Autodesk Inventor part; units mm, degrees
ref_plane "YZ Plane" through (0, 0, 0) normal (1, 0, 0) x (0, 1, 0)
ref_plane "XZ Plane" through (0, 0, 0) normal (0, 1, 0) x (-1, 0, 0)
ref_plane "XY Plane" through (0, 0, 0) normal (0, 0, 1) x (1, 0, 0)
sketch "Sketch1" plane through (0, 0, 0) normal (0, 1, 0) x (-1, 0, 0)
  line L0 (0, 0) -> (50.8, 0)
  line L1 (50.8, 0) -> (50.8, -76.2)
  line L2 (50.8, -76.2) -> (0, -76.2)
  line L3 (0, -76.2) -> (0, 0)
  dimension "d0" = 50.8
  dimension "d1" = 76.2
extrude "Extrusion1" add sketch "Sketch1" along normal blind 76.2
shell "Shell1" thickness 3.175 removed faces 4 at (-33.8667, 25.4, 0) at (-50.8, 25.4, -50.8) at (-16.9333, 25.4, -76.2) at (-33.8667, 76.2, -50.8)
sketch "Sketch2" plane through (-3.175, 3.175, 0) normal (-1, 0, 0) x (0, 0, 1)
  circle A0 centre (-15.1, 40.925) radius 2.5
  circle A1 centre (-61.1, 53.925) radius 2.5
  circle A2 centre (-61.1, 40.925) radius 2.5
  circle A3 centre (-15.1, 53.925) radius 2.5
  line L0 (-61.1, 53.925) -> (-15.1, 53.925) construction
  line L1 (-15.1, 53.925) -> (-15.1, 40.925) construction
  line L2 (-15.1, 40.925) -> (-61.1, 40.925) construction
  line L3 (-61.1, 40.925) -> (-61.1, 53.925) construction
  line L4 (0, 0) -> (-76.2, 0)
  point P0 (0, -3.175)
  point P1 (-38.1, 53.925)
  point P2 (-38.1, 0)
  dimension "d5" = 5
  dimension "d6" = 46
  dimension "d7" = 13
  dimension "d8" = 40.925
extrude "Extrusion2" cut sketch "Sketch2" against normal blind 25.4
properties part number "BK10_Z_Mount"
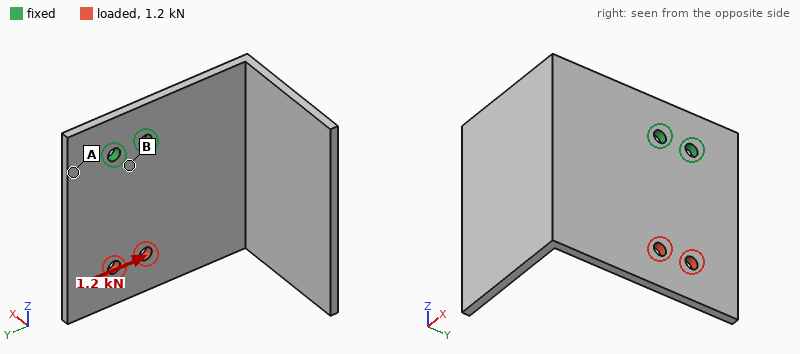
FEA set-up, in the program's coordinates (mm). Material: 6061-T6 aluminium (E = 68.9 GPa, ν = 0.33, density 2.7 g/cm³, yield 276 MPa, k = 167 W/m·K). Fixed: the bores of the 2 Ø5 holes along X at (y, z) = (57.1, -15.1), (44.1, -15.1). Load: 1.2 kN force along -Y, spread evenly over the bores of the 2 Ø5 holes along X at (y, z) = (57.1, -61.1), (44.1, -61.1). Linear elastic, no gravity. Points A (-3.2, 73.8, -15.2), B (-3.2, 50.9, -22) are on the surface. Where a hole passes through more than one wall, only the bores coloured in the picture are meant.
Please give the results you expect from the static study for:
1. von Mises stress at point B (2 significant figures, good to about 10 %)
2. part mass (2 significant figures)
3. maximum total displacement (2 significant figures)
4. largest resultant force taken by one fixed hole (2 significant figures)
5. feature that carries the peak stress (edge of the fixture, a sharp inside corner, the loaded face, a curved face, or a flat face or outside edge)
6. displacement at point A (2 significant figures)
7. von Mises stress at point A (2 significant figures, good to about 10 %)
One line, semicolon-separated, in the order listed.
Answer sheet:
58 MPa; 80 g; 0.12 mm; 3.2 kN; edge of the fixture; 0.027 mm; 14 MPa
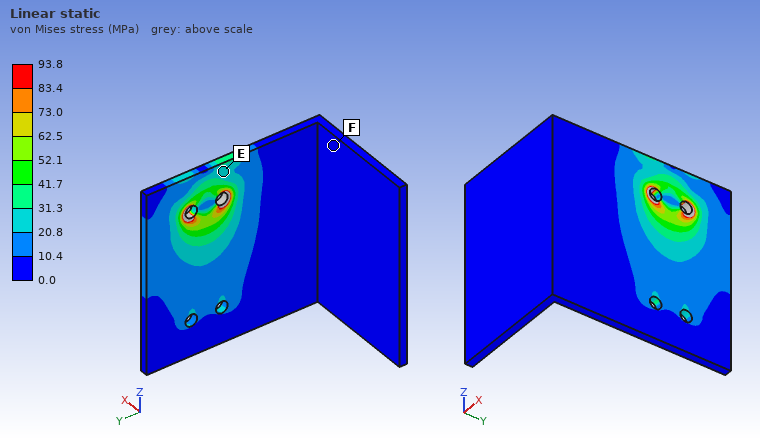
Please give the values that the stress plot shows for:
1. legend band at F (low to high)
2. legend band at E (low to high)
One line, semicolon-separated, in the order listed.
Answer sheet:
0.0 to 10.4 MPa; 20.8 to 31.3 MPa
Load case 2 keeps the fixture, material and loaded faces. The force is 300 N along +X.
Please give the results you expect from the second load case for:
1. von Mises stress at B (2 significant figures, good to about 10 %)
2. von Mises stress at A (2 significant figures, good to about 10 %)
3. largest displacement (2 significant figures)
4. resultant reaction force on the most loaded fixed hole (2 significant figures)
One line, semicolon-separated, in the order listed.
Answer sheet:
130 MPa; 50 MPa; 1.2 mm; 150 N
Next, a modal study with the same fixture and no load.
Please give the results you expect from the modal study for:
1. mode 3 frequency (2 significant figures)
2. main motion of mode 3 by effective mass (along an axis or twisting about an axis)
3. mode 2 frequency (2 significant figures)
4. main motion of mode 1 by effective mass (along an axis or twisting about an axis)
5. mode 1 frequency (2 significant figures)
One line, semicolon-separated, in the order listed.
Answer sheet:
990 Hz; along X; 460 Hz; along X; 310 Hz
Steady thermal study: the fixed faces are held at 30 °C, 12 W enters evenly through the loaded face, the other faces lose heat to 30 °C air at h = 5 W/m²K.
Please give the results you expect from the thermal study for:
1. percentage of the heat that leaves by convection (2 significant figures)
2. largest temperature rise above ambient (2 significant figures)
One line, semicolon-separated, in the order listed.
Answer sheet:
7.5 %; 21 K
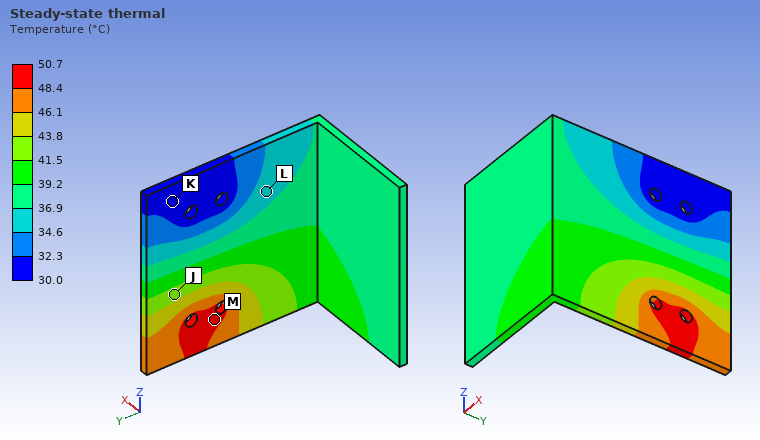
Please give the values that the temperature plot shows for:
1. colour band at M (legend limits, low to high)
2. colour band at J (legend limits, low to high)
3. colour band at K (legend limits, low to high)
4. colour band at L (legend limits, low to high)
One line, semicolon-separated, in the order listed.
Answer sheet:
48.4 to 50.7 °C; 41.5 to 43.8 °C; 30.0 to 32.3 °C; 34.6 to 36.9 °C
